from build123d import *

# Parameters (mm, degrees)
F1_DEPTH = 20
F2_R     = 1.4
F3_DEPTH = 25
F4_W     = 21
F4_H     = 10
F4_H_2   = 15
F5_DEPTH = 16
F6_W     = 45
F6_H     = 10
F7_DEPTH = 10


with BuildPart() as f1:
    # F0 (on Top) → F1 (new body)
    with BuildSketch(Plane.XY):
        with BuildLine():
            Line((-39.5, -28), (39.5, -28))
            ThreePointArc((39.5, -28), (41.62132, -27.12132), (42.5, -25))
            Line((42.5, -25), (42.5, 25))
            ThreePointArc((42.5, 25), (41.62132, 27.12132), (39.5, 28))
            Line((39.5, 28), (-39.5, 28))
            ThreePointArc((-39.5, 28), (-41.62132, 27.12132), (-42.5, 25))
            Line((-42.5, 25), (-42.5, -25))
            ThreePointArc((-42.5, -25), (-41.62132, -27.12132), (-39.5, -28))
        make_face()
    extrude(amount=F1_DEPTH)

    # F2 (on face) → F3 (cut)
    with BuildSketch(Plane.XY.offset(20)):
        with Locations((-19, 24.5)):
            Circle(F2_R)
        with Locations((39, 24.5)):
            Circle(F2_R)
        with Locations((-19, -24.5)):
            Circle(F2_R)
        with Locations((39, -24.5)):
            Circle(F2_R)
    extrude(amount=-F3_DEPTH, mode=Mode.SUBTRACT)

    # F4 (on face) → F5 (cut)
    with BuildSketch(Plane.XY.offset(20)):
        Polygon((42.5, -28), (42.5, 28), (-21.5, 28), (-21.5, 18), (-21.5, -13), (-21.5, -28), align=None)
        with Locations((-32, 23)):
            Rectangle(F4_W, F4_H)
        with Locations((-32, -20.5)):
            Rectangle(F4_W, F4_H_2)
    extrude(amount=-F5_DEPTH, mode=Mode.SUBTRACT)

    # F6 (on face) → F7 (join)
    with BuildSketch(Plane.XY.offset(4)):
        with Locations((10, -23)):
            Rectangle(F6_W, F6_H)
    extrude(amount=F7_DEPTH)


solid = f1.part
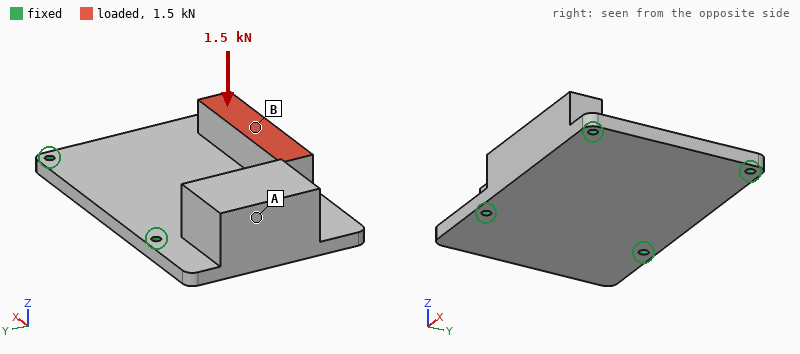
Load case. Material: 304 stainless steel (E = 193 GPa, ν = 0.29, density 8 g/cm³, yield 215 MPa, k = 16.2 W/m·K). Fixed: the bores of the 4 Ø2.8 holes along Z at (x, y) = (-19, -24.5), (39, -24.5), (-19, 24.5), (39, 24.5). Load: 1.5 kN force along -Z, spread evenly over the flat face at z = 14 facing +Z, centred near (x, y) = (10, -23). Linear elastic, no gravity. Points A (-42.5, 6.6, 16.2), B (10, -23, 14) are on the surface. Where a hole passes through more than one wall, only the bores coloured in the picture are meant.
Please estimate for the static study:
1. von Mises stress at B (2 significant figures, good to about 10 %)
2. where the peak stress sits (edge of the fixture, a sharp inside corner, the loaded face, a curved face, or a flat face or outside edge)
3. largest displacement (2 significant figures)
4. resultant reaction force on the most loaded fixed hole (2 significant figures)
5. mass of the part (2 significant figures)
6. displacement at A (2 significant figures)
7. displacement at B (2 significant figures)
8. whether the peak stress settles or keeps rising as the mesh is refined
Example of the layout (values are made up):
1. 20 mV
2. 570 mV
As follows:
1. 22 MPa
2. edge of the fixture
3. 9.8 µm
4. 900 N
5. 270 g
6. 4.6 µm
7. 9.1 µm
8. keeps rising
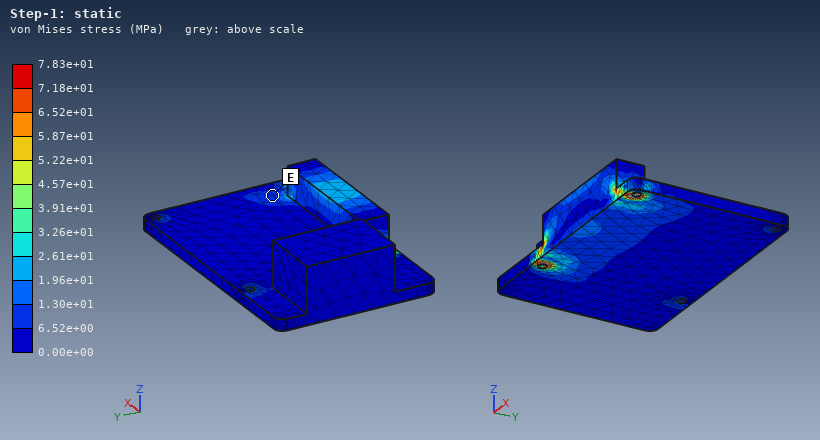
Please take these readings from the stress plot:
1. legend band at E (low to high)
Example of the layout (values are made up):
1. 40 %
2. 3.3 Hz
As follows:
1. 6.52e+00 to 1.30e+01 MPa
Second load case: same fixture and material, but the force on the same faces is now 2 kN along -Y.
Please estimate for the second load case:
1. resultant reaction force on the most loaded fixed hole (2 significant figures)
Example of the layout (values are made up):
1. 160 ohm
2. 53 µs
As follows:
1. 730 N
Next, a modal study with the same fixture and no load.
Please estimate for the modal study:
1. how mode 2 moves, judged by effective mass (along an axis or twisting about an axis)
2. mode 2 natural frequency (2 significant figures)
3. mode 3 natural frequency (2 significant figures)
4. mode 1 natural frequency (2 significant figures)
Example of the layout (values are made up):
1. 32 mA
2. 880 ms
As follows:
1. along Z
2. 4700 Hz
3. 6900 Hz
4. 2200 Hz
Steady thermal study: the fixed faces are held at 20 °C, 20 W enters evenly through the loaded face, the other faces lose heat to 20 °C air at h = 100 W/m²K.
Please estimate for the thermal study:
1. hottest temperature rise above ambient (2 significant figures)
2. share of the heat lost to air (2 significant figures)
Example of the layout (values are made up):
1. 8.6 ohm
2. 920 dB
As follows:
1. 68 K
2. 74 %
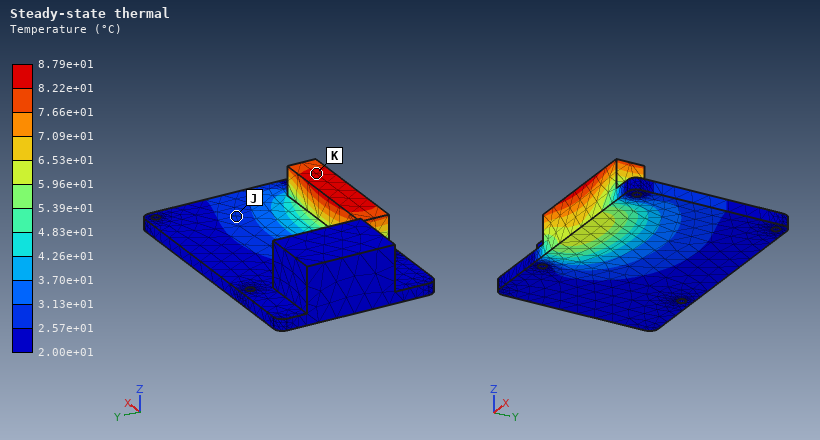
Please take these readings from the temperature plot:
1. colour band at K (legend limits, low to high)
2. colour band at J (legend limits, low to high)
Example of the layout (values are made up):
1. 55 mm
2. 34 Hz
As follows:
1. 8.22e+01 to 8.79e+01 °C
2. 2.57e+01 to 3.13e+01 °C
